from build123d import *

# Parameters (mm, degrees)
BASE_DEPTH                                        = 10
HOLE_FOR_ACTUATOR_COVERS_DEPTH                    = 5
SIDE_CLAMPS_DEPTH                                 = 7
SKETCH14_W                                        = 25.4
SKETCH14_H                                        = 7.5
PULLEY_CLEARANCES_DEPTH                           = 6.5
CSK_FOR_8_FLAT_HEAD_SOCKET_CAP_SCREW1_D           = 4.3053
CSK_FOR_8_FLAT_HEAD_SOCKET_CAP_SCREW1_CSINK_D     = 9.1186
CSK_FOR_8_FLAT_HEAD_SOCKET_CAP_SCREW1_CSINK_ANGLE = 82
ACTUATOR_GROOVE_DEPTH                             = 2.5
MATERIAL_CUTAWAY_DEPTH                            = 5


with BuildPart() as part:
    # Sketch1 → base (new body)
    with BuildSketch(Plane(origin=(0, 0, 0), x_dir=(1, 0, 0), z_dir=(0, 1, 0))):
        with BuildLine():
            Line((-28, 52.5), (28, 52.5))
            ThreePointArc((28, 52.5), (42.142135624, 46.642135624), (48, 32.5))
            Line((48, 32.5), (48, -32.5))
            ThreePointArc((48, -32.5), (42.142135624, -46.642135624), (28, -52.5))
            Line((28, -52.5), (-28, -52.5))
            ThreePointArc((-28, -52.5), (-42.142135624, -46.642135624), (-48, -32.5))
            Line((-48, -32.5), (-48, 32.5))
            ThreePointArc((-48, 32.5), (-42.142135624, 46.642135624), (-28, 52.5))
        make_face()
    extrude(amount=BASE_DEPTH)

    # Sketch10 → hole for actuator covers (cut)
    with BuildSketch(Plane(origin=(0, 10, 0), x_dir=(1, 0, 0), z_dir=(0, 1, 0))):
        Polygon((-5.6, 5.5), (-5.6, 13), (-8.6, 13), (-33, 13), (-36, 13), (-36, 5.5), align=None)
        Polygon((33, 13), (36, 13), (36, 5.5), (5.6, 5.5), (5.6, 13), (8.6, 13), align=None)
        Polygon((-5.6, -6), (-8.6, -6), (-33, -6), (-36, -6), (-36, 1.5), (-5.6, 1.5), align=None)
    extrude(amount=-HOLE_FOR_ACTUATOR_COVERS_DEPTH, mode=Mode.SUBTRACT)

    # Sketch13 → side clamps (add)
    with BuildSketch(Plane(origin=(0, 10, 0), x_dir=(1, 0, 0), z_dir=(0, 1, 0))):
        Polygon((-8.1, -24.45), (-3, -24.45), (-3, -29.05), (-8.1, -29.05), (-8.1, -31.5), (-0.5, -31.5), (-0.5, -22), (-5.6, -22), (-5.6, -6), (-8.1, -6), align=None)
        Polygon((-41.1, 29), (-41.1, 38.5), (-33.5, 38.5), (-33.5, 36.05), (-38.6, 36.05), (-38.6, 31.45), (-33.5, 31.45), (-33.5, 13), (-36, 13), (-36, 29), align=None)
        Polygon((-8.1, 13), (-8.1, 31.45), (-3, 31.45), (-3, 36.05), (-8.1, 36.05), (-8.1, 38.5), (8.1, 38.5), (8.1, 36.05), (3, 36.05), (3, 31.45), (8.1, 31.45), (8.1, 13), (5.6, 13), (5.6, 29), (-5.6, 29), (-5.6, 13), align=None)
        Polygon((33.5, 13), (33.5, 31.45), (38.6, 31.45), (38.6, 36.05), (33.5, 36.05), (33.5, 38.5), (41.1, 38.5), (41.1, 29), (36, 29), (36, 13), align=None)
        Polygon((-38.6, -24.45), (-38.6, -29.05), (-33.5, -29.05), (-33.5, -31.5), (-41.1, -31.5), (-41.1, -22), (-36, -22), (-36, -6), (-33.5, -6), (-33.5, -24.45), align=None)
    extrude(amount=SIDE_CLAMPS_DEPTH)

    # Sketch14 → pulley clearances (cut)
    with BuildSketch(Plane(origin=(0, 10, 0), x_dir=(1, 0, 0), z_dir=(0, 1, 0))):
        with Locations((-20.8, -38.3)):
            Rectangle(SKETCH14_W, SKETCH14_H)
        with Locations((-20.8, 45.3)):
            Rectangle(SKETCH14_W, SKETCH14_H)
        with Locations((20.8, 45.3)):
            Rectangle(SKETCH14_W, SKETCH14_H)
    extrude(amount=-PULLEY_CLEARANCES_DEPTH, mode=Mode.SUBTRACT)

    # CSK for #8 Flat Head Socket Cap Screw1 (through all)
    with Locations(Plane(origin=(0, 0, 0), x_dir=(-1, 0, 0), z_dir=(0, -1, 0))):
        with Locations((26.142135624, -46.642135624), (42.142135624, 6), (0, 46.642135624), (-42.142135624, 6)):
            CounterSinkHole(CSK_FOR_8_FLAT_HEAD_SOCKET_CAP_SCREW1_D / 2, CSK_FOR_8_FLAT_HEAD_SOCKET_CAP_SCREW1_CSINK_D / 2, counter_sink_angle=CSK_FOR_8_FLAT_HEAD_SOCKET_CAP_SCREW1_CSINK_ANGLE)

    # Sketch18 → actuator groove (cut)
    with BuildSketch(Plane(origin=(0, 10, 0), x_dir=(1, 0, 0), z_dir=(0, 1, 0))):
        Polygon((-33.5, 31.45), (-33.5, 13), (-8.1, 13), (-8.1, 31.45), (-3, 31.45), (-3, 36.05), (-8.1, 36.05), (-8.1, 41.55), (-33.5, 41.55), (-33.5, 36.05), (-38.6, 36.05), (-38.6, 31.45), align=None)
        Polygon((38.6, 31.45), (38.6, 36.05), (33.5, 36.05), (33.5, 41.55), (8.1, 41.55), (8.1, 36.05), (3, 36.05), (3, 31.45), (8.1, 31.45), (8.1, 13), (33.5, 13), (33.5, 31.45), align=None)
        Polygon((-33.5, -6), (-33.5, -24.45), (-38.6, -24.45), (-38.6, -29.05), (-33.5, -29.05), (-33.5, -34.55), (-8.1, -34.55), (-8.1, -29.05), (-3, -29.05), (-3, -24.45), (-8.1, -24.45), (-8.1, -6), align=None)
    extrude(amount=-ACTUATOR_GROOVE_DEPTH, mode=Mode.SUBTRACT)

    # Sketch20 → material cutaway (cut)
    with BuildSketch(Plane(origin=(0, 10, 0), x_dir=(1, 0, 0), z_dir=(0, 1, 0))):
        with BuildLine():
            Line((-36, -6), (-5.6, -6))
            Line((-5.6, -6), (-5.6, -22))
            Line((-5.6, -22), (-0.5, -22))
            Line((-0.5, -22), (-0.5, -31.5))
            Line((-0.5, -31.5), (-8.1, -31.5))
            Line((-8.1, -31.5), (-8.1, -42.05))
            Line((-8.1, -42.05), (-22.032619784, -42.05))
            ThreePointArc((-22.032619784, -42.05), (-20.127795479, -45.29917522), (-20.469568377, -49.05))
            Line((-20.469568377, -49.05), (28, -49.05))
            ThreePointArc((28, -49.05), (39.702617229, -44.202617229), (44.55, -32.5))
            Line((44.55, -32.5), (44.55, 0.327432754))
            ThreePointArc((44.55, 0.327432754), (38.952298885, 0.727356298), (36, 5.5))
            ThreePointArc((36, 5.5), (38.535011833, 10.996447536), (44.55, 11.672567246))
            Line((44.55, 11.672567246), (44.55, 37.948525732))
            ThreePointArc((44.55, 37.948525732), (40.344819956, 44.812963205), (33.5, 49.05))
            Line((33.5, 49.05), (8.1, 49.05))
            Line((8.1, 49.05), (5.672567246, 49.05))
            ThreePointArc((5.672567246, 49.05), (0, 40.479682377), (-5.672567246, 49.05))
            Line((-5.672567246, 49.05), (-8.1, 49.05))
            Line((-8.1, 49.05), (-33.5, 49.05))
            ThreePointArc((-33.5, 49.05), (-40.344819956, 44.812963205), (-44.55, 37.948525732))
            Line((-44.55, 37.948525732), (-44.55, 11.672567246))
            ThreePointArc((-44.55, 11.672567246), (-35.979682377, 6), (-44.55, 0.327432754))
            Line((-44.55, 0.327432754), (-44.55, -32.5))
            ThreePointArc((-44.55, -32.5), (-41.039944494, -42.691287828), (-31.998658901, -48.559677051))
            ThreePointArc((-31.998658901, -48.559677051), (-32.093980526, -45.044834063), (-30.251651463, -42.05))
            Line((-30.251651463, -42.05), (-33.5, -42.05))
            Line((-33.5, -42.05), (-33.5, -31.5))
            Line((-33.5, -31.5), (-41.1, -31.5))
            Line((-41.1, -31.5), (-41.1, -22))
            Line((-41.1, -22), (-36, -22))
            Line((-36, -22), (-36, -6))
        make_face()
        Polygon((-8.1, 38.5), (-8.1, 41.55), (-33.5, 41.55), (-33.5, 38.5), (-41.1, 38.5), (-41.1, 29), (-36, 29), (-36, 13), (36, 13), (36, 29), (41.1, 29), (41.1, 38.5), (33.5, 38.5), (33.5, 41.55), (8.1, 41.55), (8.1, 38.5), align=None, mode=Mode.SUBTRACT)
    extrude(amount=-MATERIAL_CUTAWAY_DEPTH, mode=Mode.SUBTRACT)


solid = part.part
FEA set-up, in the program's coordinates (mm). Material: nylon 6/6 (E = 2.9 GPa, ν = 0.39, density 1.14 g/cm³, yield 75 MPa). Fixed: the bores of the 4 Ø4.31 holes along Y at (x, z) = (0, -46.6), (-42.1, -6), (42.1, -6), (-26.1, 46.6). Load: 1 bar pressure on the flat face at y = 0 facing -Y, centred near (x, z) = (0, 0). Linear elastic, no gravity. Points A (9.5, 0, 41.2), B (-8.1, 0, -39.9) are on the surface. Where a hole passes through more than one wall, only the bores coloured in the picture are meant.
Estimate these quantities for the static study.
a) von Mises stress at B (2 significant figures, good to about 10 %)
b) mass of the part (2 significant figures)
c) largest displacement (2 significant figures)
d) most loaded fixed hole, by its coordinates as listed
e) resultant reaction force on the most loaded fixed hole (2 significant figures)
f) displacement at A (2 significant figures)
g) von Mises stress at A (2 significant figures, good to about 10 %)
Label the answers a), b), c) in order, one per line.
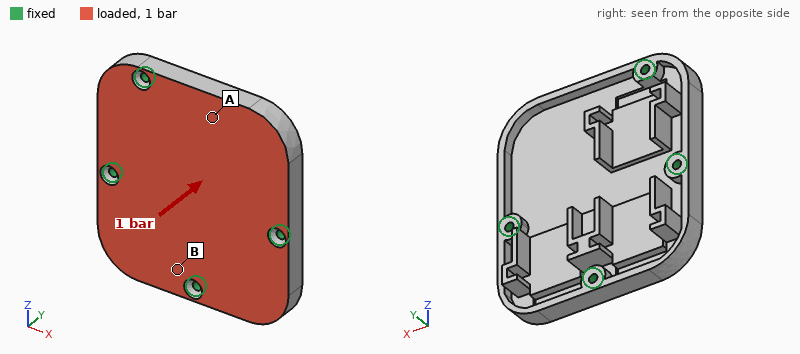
a) 3.2 MPa
b) 77 g
c) 0.98 mm
d) (42.1, -6)
e) 370 N
f) 0.53 mm
g) 6.0 MPa
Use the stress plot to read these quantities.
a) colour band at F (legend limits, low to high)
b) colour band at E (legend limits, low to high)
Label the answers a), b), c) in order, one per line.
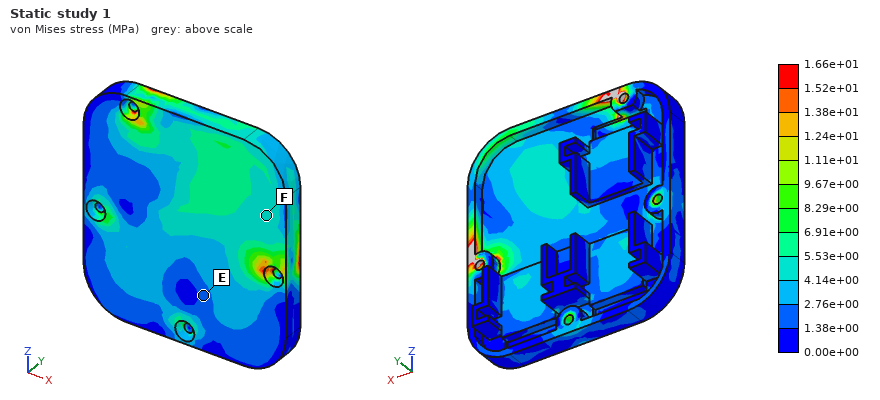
a) 4.14e+00 to 5.53e+00 MPa
b) 1.38e+00 to 2.76e+00 MPa
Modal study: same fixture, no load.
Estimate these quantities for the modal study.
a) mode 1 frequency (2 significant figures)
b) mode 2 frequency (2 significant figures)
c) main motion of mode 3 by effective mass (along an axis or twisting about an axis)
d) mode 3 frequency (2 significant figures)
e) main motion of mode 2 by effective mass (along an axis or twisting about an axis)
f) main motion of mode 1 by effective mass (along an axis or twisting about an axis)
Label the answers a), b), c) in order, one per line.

a) 810 Hz
b) 1400 Hz
c) twisting about Z
d) 1600 Hz
e) along Y
f) along Y
